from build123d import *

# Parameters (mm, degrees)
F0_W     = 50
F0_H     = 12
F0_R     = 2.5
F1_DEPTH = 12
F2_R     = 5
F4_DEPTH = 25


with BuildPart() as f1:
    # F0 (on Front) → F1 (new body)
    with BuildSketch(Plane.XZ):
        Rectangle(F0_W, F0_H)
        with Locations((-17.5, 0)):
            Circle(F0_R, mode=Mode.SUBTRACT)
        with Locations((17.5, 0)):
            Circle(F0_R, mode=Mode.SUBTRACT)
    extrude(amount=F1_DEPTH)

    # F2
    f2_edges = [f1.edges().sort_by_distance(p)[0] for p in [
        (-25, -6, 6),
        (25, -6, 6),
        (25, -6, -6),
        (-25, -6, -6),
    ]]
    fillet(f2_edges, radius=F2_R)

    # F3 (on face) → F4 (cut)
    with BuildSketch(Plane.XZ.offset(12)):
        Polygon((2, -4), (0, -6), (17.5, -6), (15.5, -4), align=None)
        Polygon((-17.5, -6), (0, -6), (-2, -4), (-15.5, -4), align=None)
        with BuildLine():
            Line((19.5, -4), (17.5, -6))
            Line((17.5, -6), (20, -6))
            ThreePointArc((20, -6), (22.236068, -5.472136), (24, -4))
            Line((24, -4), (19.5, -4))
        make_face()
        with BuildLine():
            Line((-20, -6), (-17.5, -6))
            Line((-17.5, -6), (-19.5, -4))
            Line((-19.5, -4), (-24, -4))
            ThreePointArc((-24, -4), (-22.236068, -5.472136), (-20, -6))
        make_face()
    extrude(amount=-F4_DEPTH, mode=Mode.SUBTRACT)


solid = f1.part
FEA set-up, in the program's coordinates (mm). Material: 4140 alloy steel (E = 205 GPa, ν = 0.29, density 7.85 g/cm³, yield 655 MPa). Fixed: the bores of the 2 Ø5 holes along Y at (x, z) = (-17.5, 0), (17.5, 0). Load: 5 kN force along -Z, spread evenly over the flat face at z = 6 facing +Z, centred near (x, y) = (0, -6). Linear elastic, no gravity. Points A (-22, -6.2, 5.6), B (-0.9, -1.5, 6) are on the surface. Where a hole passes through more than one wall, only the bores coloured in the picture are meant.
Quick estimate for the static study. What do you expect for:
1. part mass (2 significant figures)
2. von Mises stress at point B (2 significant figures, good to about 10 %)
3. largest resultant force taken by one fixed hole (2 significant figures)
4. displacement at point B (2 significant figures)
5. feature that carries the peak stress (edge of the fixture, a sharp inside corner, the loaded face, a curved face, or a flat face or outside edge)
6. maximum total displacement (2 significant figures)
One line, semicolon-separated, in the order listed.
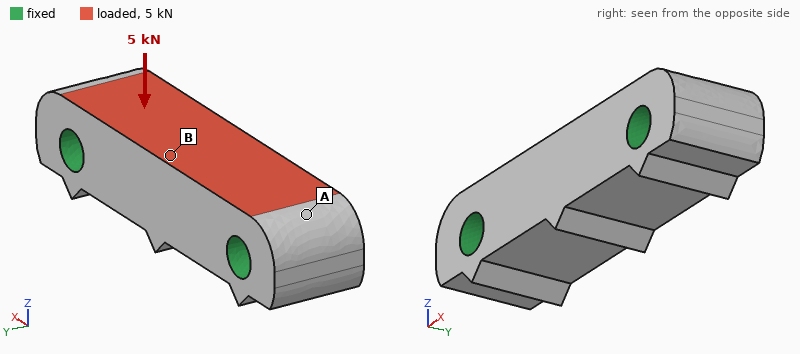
43 g; 35 MPa; 2.5 kN; 4.4 µm; edge of the fixture; 4.5 µm
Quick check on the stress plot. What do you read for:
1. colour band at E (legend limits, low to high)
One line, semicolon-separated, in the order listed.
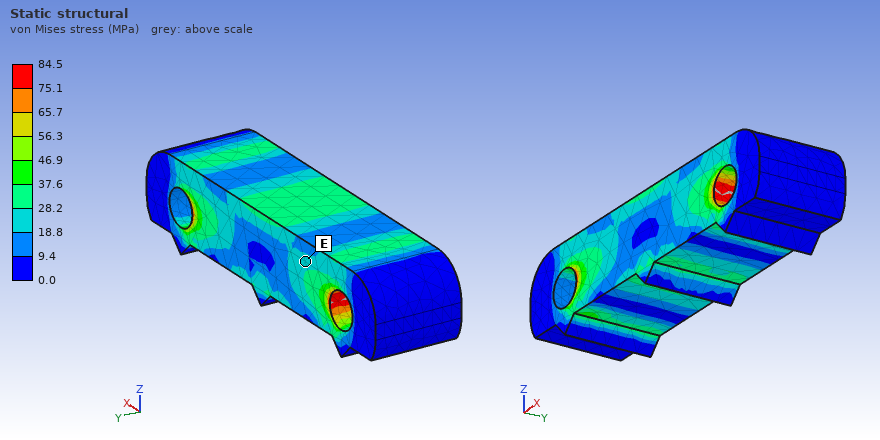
18.8 to 28.2 MPa
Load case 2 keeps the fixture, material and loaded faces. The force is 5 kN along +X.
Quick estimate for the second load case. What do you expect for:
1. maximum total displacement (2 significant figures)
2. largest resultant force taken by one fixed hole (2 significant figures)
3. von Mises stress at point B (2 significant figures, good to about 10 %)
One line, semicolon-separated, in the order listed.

1.2 µm; 2.6 kN; 18 MPa
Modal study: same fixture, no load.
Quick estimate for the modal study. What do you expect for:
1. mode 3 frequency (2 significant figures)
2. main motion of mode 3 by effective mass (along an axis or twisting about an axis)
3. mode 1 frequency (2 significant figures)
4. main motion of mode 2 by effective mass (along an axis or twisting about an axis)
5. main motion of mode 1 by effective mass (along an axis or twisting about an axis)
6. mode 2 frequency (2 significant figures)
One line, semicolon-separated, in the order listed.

44 kHz; twisting about X; 31 kHz; along Y; along Z; 36 kHz
